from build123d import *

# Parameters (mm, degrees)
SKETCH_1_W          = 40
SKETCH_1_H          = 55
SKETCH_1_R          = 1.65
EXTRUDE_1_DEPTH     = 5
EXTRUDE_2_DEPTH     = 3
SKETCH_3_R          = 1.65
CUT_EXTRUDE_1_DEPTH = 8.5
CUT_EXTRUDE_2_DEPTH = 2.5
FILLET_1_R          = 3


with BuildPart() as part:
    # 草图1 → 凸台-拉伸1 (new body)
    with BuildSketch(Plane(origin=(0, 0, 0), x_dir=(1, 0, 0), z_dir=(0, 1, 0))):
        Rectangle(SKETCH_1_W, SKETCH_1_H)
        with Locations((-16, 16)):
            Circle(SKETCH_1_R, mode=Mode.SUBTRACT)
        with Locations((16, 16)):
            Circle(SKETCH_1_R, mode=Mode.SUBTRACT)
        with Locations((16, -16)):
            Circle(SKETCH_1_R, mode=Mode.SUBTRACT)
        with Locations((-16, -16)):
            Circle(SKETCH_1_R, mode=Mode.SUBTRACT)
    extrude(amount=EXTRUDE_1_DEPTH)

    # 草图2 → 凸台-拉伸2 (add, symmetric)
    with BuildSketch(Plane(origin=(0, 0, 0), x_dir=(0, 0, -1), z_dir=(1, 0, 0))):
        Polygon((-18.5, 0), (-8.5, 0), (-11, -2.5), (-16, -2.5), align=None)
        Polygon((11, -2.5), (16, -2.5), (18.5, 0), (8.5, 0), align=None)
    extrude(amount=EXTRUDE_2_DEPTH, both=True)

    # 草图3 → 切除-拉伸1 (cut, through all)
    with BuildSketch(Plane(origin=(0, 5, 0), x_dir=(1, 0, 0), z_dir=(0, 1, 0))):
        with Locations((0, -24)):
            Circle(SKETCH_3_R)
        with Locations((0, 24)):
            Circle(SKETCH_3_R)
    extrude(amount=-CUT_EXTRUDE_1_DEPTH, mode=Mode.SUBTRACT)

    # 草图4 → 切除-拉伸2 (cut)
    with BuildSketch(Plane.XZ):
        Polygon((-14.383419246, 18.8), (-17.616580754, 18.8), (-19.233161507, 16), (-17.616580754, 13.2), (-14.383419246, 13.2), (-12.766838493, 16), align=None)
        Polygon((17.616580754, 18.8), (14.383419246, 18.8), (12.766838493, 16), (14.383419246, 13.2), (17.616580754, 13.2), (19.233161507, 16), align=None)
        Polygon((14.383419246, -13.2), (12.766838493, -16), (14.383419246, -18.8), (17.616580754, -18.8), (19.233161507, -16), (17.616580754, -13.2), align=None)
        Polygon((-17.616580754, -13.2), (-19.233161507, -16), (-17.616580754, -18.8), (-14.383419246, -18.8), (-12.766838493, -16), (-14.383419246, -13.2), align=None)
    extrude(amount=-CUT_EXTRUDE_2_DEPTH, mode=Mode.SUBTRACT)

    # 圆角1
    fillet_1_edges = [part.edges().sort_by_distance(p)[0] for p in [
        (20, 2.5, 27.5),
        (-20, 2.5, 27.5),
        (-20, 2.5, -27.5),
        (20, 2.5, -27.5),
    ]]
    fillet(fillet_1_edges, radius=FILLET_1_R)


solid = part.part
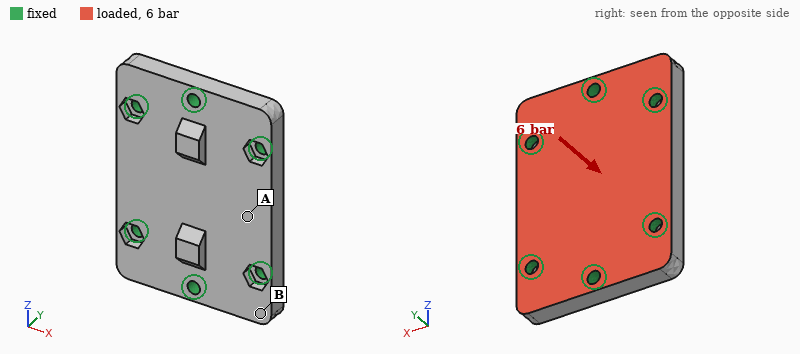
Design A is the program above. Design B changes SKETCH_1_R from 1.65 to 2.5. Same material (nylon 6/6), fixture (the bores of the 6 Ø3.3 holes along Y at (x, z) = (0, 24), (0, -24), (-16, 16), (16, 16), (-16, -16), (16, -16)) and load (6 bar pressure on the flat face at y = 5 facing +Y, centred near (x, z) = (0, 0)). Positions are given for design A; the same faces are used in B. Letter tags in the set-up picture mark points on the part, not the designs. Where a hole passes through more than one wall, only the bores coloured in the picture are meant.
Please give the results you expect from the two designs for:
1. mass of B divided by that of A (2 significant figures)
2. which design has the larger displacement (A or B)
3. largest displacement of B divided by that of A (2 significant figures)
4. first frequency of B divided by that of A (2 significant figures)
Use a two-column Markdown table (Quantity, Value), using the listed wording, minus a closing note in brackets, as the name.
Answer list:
| Quantity | Value |
|---|---|
| mass of B divided by that of A | 0.99 |
| which design has the larger displacement | A |
| largest displacement of B divided by that of A | 0.83 |
| first frequency of B divided by that of A | 1.1 |
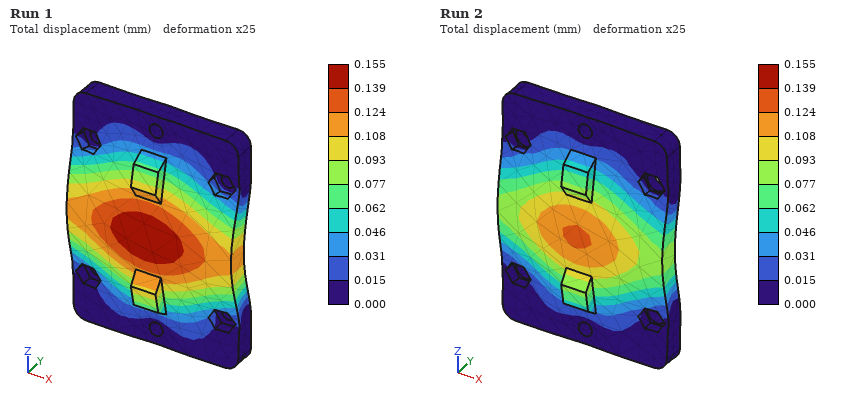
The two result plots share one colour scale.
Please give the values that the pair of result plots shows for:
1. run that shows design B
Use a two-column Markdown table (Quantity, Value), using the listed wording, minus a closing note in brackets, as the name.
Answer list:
| Quantity | Value |
|---|---|
| run that shows design B | Run 2 |
